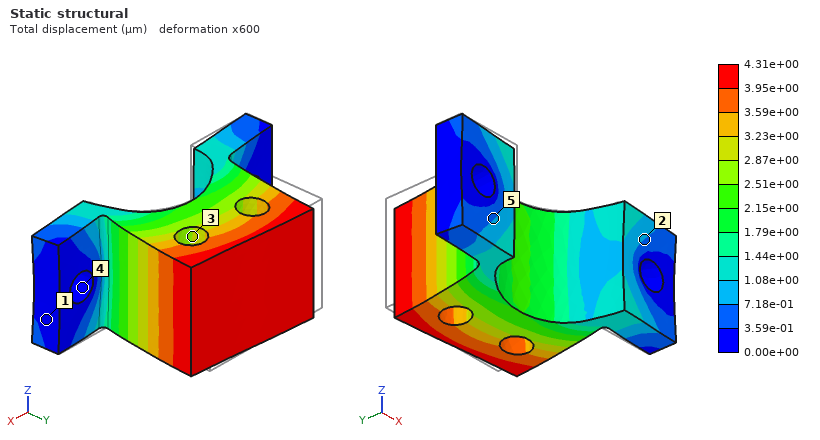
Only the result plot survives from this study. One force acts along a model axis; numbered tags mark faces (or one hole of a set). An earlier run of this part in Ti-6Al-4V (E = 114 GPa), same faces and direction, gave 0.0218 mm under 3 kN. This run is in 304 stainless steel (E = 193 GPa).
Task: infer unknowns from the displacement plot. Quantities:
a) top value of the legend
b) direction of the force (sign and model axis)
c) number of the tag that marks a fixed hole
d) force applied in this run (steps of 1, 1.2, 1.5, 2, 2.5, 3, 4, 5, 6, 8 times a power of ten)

4.31e+00 µm
+X
4
1 kN
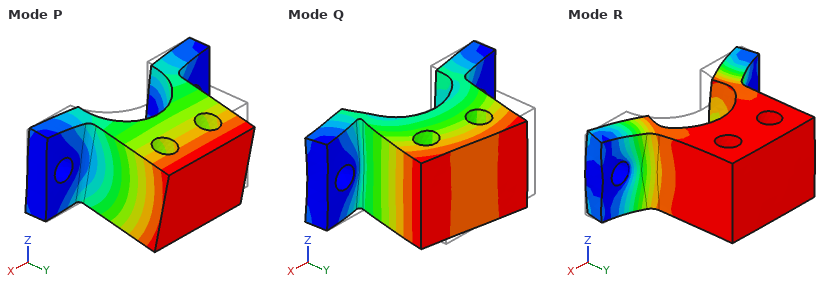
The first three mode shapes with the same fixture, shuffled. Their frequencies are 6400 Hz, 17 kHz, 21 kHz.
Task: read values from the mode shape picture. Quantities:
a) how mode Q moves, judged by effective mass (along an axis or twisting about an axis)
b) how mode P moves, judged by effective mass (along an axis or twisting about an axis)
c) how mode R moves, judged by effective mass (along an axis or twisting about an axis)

along X
along Z
along Y
